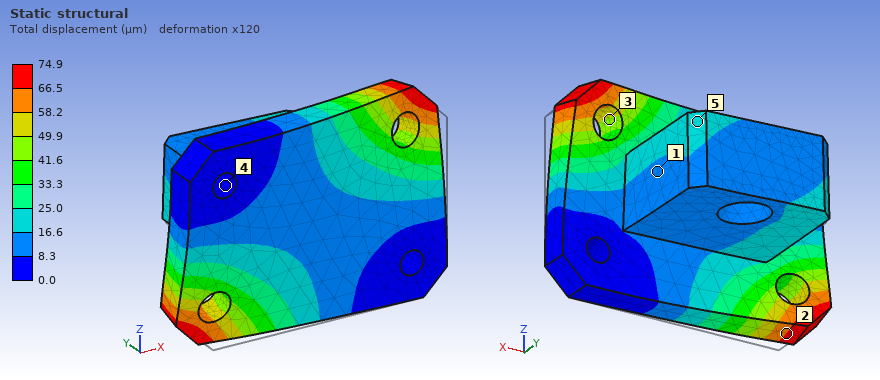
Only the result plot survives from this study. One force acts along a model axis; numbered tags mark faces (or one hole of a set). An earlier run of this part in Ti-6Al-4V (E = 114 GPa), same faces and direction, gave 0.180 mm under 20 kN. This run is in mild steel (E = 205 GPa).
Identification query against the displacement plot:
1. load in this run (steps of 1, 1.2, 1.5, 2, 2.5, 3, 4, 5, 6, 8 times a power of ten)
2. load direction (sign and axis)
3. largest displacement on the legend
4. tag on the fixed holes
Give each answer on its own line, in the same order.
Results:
15 kN
+Y
74.9 µm
4
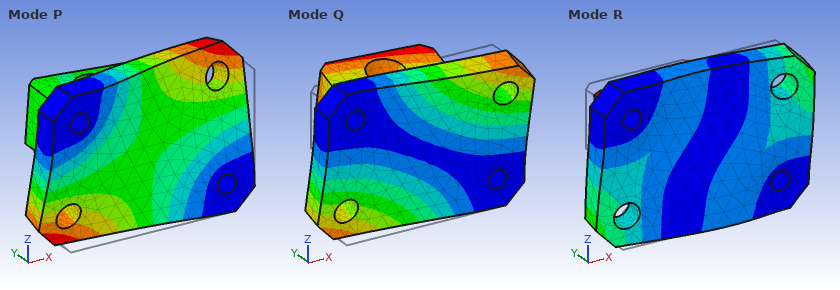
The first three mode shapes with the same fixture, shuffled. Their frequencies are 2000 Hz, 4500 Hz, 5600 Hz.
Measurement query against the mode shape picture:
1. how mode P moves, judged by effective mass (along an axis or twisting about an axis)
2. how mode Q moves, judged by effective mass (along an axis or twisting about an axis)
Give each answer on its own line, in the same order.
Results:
along Y
along Z
